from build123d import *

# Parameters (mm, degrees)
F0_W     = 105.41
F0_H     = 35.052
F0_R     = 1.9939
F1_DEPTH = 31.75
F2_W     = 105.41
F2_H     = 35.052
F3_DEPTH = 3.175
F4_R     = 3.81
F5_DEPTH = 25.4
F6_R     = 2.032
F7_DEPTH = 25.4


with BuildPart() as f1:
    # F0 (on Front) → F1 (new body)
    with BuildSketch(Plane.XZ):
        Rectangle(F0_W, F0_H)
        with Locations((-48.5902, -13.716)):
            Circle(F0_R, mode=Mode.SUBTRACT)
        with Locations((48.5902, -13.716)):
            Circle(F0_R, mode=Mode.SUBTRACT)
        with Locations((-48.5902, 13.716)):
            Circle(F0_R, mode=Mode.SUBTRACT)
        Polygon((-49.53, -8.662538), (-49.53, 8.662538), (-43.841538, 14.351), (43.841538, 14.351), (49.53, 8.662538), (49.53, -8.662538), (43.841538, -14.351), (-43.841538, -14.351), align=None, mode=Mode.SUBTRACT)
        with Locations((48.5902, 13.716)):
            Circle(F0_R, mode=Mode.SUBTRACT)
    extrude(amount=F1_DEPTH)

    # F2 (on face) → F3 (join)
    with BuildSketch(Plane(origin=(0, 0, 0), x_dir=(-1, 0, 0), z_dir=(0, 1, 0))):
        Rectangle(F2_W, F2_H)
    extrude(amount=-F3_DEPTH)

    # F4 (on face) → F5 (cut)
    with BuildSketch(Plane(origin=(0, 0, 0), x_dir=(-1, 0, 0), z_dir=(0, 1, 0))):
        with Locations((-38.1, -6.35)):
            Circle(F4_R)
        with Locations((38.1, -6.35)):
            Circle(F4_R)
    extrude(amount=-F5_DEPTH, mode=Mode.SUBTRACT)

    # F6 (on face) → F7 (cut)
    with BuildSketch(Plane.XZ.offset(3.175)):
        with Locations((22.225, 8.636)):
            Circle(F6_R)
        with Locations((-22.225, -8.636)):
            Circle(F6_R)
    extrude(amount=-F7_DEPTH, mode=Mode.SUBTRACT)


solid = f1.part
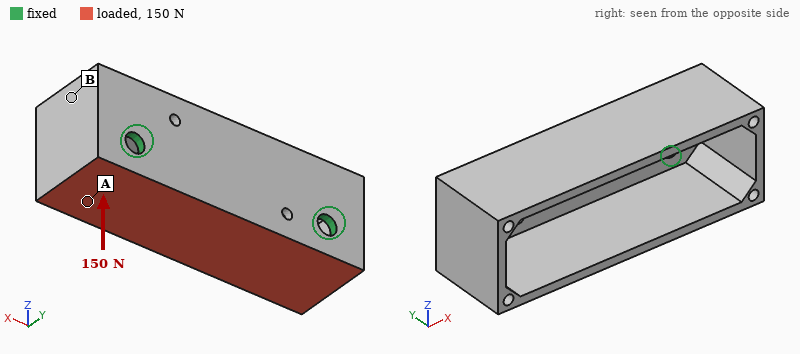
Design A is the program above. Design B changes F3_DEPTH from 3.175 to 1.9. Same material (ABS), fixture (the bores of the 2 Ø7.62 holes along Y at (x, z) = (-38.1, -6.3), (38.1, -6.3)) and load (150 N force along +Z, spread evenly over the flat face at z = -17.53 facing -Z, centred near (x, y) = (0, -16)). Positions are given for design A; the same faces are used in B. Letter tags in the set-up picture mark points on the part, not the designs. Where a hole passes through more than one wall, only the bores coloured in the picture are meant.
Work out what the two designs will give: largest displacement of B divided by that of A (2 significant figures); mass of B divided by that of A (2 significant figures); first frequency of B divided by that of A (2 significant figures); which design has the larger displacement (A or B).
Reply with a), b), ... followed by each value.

a) 2.2
b) 0.90
c) 0.55
d) B
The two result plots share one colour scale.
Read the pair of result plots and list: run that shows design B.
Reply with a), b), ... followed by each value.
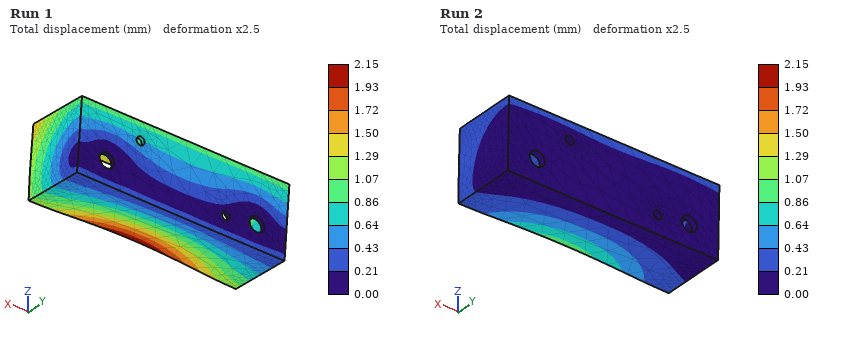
a) Run 1
